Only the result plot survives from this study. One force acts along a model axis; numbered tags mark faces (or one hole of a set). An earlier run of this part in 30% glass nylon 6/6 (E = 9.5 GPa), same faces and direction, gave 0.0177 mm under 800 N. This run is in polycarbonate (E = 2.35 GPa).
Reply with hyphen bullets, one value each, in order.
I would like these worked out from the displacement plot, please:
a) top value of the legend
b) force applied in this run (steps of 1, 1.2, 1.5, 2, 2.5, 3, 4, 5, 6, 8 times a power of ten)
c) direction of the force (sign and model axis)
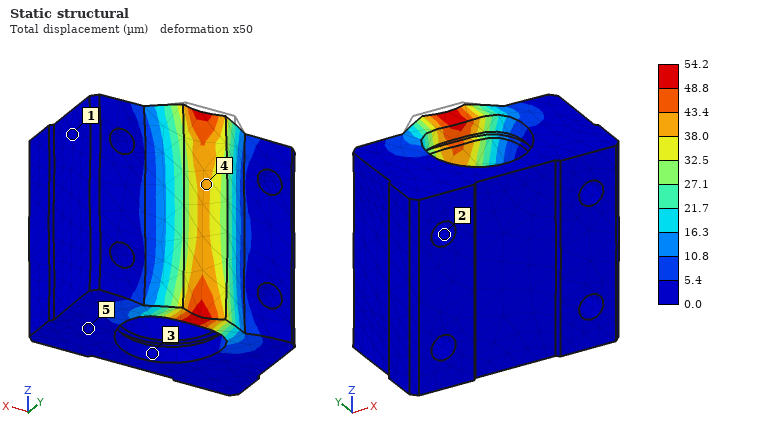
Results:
- 54.2 µm
- 600 N
- -Y
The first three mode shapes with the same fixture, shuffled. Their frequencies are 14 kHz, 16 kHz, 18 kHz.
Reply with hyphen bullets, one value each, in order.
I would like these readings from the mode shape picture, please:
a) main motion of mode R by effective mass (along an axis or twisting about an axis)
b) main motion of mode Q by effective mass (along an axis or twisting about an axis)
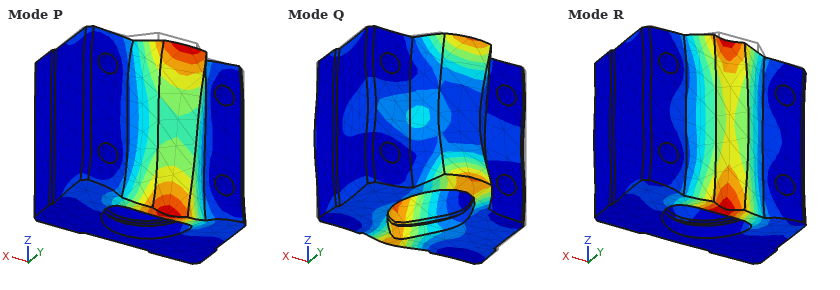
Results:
- along Y
- along Y
